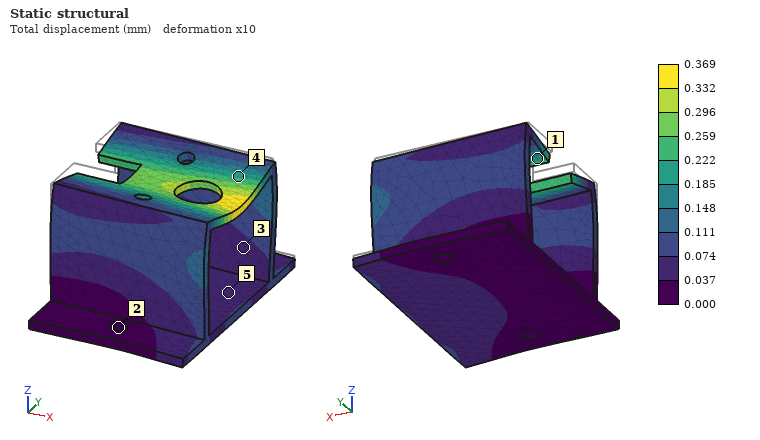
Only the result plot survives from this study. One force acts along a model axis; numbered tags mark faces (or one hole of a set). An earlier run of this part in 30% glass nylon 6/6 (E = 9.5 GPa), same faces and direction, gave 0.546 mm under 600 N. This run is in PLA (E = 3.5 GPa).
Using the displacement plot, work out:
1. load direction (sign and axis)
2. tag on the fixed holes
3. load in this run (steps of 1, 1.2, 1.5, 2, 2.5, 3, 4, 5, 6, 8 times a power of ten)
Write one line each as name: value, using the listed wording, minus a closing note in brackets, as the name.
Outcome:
load direction: -Z
tag on the fixed holes: 2
load in this run: 150 N
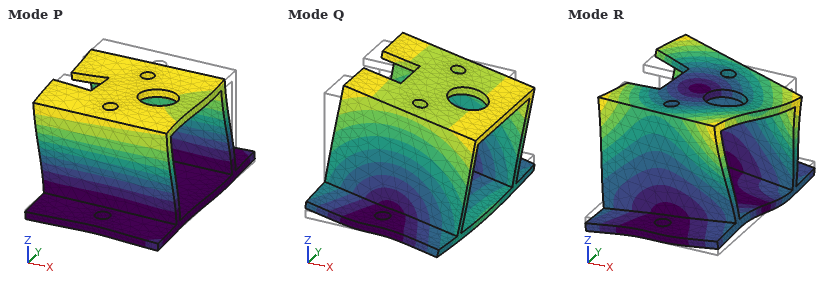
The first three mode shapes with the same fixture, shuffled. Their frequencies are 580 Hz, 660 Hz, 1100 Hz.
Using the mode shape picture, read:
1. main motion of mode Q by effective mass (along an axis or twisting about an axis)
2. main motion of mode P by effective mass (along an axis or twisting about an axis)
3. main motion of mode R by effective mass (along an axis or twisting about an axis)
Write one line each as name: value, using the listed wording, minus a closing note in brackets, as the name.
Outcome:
main motion of mode Q by effective mass: along X
main motion of mode P by effective mass: along Y
main motion of mode R by effective mass: twisting about Z
